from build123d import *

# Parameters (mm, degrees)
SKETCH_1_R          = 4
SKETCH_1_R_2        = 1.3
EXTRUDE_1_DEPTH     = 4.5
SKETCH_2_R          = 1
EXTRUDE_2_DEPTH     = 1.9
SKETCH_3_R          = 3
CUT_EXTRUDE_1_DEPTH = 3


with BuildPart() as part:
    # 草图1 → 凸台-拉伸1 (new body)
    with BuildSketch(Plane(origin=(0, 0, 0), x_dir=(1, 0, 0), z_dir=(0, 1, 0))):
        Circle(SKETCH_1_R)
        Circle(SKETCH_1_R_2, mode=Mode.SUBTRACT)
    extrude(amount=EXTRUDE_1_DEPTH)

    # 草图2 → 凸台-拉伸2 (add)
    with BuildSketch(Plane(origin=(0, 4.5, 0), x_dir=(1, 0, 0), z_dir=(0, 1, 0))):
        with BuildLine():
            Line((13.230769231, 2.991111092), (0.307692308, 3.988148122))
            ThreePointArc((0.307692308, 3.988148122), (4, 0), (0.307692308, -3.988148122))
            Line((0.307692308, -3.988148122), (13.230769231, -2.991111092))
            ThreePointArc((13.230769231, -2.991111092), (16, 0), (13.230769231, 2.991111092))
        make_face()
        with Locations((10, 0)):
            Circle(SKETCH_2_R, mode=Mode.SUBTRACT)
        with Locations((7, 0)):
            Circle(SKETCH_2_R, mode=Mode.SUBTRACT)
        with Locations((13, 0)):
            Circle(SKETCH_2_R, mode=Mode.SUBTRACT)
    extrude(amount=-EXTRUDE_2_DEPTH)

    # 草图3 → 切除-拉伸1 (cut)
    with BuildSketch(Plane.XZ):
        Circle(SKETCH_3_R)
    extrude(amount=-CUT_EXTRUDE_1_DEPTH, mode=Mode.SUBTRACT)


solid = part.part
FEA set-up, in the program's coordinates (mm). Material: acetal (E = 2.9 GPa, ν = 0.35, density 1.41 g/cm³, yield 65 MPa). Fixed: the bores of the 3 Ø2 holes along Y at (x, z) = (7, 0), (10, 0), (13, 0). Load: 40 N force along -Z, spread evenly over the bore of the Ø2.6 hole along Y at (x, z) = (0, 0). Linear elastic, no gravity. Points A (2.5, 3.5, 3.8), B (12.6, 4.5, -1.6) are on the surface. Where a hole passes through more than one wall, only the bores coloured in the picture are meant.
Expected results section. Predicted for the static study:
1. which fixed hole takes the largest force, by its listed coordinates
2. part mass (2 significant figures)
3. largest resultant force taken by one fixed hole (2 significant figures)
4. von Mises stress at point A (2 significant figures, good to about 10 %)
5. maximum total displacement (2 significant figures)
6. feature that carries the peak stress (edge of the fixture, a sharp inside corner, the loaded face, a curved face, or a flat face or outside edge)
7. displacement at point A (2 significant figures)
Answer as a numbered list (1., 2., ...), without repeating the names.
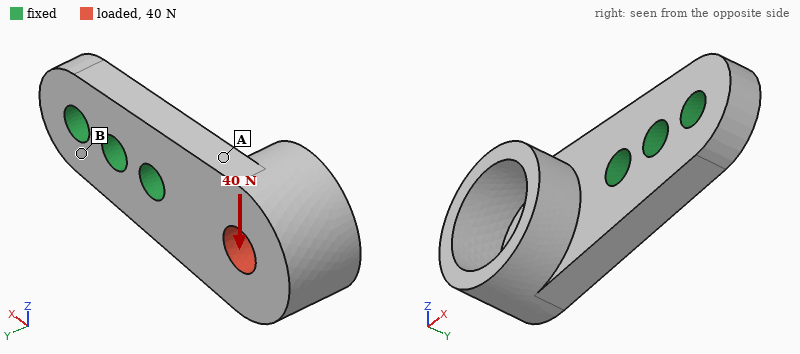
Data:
1. (7, 0)
2. 0.38 g
3. 72 N
4. 7.3 MPa
5. 0.12 mm
6. edge of the fixture
7. 0.058 mm
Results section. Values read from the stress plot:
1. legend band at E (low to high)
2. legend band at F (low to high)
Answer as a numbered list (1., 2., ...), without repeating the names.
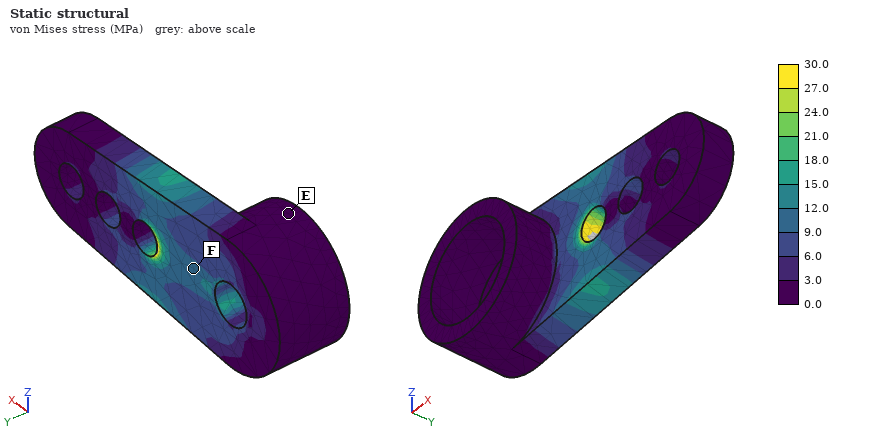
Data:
1. 0.0 to 3.0 MPa
2. 9.0 to 12.0 MPa
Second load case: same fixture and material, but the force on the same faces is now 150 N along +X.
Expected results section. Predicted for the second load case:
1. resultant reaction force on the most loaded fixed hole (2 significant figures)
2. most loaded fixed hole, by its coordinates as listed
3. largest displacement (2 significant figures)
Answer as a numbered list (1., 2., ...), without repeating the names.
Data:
1. 120 N
2. (7, 0)
3. 0.12 mm
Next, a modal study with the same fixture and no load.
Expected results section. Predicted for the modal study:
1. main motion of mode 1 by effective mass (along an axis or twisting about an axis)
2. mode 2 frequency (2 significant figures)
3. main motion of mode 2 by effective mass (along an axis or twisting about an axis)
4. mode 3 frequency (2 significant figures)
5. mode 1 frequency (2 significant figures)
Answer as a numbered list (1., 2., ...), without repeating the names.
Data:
1. along Y
2. 6700 Hz
3. along Z
4. 8700 Hz
5. 3400 Hz
